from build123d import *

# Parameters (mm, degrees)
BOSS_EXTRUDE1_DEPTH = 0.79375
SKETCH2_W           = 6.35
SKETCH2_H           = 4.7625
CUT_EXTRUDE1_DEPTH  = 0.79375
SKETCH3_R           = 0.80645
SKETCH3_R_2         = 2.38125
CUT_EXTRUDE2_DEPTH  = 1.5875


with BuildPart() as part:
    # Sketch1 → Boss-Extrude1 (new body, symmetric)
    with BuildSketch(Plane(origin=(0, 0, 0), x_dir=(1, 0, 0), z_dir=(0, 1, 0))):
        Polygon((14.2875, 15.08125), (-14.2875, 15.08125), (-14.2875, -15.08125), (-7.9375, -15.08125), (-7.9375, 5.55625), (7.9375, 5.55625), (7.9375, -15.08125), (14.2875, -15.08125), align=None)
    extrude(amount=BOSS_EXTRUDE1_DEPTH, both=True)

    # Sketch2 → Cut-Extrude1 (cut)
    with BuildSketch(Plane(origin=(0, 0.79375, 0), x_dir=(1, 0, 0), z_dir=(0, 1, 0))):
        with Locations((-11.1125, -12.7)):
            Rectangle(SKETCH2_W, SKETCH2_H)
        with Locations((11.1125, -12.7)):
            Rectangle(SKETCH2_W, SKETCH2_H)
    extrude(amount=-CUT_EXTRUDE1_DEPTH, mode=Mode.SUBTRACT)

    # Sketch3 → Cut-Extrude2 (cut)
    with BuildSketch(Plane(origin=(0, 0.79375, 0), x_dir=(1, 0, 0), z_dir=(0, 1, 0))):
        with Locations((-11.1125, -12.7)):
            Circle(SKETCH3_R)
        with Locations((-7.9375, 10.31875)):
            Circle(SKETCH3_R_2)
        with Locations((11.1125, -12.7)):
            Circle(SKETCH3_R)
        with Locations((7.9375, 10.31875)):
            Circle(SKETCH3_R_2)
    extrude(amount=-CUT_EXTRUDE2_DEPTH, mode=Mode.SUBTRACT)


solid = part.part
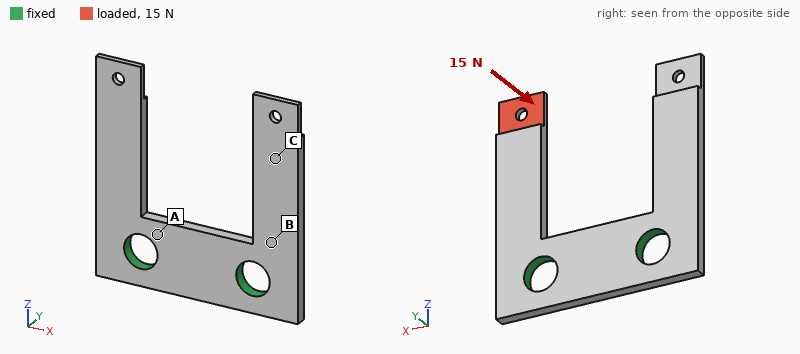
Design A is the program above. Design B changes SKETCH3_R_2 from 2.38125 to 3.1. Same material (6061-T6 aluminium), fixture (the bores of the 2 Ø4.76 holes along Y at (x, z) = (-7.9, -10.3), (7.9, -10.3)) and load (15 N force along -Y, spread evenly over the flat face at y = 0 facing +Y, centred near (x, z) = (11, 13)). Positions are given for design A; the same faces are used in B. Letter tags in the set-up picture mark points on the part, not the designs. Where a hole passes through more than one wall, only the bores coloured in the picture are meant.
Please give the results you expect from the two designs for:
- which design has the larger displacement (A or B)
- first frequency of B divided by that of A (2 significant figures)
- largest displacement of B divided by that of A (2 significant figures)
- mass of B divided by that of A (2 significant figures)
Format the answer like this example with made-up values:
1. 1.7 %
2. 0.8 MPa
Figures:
1. A
2. 1.1
3. 0.92
4. 0.95
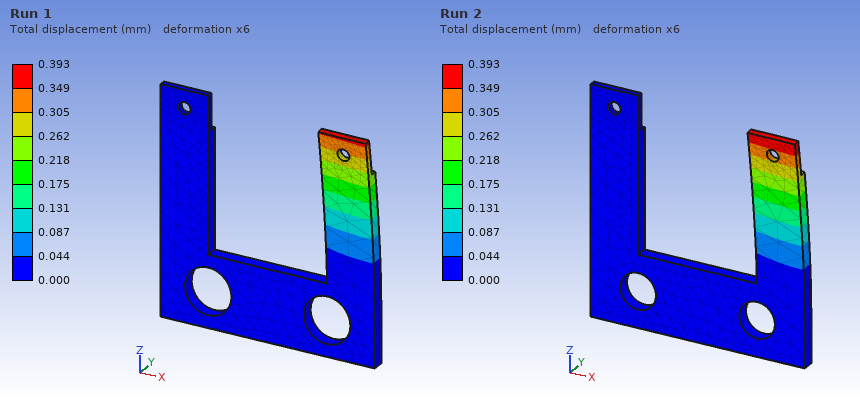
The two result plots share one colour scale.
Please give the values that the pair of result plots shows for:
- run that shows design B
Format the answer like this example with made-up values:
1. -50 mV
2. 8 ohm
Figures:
1. Run 1
